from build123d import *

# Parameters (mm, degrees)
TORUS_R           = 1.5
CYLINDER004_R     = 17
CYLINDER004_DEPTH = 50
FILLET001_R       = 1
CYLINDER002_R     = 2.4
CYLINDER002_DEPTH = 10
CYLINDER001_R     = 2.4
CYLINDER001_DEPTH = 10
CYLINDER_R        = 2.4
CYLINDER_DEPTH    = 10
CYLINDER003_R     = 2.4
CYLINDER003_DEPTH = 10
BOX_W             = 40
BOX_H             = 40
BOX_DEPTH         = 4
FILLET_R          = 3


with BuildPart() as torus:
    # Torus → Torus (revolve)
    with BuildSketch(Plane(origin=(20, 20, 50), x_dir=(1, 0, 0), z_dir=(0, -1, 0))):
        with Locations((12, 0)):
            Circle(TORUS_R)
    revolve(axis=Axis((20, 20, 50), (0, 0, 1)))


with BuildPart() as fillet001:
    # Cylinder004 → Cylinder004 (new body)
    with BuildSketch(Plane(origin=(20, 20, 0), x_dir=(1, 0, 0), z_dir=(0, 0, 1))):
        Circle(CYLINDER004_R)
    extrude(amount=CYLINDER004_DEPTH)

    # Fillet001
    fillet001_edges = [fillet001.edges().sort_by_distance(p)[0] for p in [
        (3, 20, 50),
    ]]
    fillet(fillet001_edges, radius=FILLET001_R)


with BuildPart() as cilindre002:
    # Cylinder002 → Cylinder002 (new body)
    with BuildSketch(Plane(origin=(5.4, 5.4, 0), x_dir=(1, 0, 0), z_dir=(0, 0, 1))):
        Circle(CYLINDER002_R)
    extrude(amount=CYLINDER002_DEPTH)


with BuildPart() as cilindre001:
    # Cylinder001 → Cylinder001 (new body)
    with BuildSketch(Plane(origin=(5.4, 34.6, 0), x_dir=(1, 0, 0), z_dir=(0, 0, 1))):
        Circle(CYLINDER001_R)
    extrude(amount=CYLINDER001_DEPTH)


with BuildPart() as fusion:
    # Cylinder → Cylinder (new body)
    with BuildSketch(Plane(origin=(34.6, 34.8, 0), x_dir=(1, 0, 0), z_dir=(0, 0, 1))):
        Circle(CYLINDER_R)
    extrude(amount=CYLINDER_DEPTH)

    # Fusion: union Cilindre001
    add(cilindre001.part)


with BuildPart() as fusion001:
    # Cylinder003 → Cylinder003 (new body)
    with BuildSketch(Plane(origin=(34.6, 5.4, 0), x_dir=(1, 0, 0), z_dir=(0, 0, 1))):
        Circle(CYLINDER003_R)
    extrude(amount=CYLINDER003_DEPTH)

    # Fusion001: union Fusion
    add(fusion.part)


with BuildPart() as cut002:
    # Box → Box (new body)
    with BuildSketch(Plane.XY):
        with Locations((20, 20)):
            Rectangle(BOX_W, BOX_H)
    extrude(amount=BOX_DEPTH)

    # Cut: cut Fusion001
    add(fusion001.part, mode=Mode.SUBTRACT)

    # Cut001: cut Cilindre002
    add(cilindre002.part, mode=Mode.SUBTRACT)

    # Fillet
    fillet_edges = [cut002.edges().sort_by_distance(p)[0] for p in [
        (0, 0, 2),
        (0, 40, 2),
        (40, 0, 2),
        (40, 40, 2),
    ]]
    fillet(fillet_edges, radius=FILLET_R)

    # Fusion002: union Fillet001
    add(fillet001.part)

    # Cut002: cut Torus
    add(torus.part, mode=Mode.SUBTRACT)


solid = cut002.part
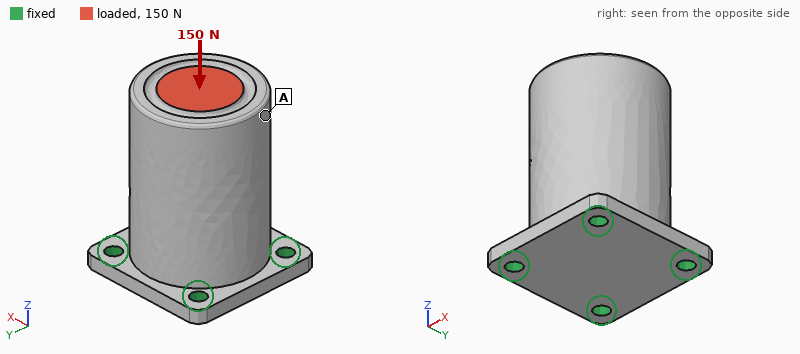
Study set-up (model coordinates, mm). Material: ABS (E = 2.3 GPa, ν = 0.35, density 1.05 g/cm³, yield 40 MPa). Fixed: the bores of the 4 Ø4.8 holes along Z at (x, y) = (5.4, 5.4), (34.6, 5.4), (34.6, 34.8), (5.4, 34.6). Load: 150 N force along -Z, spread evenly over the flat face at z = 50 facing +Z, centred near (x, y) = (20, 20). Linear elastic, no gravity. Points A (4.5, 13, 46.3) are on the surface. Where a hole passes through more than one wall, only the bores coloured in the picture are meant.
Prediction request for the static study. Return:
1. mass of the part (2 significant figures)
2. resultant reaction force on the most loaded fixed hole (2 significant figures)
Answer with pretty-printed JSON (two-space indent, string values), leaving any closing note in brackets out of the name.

{
  "mass of the part": "50 g",
  "resultant reaction force on the most loaded fixed hole": "41 N"
}
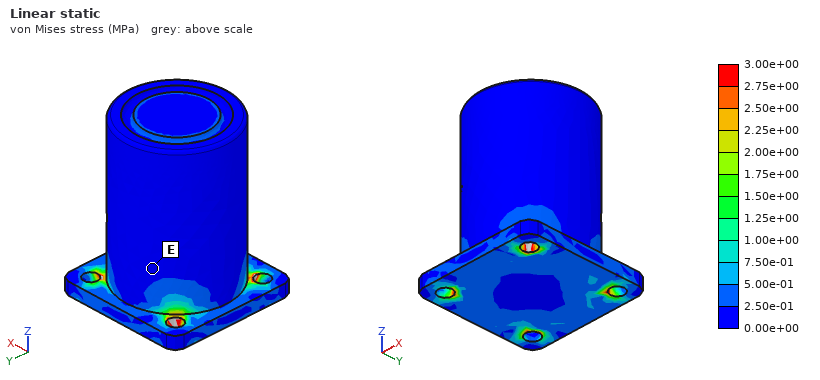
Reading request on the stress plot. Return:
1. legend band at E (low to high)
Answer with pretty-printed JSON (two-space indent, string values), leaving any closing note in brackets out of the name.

{
  "legend band at E": "0.00e+00 to 2.50e-01 MPa"
}
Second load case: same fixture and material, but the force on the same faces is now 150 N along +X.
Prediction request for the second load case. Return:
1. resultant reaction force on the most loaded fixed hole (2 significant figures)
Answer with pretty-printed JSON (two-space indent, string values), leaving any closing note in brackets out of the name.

{
  "resultant reaction force on the most loaded fixed hole": "150 N"
}
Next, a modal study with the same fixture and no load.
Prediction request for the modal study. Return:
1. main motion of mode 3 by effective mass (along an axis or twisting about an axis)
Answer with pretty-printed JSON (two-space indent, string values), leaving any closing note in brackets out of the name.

{
  "main motion of mode 3 by effective mass": "along Z"
}
